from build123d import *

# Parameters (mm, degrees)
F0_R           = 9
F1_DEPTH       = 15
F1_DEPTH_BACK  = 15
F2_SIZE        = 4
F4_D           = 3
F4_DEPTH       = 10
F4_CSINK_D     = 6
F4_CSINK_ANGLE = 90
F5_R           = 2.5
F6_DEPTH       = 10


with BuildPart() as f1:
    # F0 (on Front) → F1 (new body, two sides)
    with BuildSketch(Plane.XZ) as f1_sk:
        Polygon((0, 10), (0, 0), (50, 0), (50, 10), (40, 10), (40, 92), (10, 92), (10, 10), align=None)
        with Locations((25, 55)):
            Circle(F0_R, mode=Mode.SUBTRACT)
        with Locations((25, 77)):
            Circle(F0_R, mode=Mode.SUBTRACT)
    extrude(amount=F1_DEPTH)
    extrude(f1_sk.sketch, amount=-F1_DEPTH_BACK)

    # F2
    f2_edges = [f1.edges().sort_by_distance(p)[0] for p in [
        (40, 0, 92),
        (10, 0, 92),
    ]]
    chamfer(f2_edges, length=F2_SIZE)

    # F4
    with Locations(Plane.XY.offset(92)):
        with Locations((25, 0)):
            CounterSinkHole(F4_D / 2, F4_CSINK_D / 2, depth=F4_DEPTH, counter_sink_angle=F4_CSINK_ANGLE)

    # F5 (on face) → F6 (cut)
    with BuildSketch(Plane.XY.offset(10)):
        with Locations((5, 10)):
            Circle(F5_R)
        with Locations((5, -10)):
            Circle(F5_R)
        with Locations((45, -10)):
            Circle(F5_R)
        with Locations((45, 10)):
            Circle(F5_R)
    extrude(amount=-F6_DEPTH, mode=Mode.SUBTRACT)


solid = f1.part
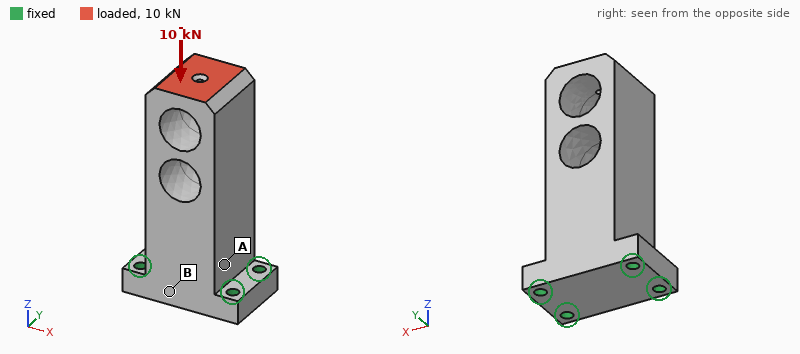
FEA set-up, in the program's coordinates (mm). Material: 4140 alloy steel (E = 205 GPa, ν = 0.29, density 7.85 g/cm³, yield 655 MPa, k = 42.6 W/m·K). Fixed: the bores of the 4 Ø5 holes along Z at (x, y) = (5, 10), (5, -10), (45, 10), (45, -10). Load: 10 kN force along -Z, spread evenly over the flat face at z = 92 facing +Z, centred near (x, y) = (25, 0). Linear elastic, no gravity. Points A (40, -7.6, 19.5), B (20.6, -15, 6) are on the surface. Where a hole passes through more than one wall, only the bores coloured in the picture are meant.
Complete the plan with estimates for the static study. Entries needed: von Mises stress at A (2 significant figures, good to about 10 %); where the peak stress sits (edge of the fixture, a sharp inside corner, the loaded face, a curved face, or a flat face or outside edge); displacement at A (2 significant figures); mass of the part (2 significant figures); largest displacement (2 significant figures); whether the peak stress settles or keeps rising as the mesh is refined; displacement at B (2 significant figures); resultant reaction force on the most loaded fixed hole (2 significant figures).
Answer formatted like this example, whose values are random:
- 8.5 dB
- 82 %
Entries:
- 15 MPa
- edge of the fixture
- 3.1 µm
- 570 g
- 15 µm
- keeps rising
- 3.0 µm
- 2.7 kN
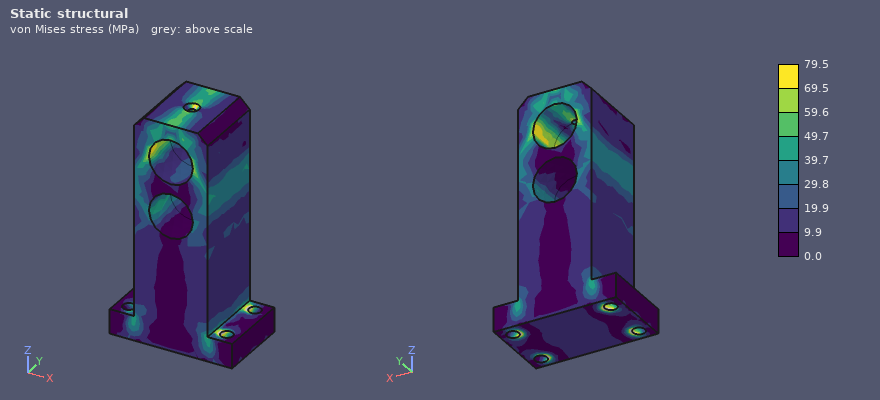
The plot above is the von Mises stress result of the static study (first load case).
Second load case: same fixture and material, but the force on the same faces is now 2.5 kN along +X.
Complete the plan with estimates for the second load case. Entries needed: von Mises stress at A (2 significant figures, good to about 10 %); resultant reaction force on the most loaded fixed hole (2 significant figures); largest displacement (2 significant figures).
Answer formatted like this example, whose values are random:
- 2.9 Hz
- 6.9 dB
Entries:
- 42 MPa
- 3.3 kN
- 68 µm
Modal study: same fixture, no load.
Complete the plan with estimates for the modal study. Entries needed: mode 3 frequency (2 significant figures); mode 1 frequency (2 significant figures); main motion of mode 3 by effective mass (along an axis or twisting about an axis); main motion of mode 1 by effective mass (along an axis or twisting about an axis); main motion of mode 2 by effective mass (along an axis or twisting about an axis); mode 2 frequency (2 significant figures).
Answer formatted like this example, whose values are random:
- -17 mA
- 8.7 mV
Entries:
- 7700 Hz
- 2400 Hz
- twisting about Z
- along Y
- along X
- 3000 Hz
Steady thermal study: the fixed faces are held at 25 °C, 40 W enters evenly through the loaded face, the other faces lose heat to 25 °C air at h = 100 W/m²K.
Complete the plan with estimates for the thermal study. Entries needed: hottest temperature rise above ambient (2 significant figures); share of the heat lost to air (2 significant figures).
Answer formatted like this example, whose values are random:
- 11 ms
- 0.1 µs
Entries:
- 70 K
- 80 %
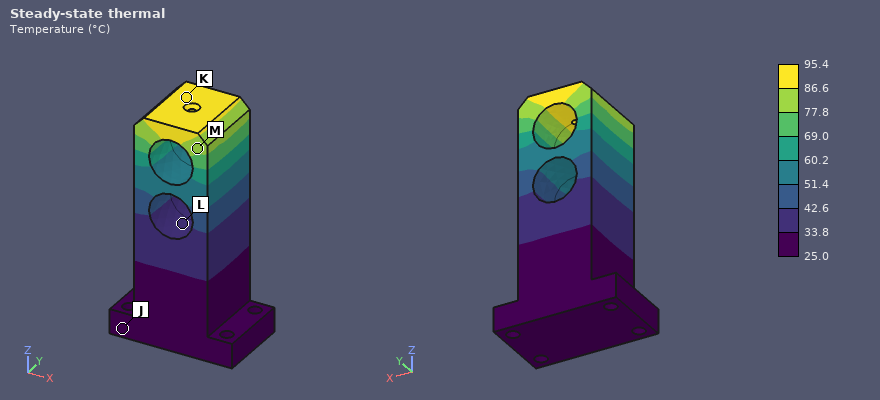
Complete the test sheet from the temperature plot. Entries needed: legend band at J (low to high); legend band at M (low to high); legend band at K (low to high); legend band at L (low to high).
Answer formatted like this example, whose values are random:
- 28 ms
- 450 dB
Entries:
- 25.0 to 33.8 °C
- 77.8 to 86.6 °C
- 86.6 to 95.4 °C
- 33.8 to 42.6 °C
